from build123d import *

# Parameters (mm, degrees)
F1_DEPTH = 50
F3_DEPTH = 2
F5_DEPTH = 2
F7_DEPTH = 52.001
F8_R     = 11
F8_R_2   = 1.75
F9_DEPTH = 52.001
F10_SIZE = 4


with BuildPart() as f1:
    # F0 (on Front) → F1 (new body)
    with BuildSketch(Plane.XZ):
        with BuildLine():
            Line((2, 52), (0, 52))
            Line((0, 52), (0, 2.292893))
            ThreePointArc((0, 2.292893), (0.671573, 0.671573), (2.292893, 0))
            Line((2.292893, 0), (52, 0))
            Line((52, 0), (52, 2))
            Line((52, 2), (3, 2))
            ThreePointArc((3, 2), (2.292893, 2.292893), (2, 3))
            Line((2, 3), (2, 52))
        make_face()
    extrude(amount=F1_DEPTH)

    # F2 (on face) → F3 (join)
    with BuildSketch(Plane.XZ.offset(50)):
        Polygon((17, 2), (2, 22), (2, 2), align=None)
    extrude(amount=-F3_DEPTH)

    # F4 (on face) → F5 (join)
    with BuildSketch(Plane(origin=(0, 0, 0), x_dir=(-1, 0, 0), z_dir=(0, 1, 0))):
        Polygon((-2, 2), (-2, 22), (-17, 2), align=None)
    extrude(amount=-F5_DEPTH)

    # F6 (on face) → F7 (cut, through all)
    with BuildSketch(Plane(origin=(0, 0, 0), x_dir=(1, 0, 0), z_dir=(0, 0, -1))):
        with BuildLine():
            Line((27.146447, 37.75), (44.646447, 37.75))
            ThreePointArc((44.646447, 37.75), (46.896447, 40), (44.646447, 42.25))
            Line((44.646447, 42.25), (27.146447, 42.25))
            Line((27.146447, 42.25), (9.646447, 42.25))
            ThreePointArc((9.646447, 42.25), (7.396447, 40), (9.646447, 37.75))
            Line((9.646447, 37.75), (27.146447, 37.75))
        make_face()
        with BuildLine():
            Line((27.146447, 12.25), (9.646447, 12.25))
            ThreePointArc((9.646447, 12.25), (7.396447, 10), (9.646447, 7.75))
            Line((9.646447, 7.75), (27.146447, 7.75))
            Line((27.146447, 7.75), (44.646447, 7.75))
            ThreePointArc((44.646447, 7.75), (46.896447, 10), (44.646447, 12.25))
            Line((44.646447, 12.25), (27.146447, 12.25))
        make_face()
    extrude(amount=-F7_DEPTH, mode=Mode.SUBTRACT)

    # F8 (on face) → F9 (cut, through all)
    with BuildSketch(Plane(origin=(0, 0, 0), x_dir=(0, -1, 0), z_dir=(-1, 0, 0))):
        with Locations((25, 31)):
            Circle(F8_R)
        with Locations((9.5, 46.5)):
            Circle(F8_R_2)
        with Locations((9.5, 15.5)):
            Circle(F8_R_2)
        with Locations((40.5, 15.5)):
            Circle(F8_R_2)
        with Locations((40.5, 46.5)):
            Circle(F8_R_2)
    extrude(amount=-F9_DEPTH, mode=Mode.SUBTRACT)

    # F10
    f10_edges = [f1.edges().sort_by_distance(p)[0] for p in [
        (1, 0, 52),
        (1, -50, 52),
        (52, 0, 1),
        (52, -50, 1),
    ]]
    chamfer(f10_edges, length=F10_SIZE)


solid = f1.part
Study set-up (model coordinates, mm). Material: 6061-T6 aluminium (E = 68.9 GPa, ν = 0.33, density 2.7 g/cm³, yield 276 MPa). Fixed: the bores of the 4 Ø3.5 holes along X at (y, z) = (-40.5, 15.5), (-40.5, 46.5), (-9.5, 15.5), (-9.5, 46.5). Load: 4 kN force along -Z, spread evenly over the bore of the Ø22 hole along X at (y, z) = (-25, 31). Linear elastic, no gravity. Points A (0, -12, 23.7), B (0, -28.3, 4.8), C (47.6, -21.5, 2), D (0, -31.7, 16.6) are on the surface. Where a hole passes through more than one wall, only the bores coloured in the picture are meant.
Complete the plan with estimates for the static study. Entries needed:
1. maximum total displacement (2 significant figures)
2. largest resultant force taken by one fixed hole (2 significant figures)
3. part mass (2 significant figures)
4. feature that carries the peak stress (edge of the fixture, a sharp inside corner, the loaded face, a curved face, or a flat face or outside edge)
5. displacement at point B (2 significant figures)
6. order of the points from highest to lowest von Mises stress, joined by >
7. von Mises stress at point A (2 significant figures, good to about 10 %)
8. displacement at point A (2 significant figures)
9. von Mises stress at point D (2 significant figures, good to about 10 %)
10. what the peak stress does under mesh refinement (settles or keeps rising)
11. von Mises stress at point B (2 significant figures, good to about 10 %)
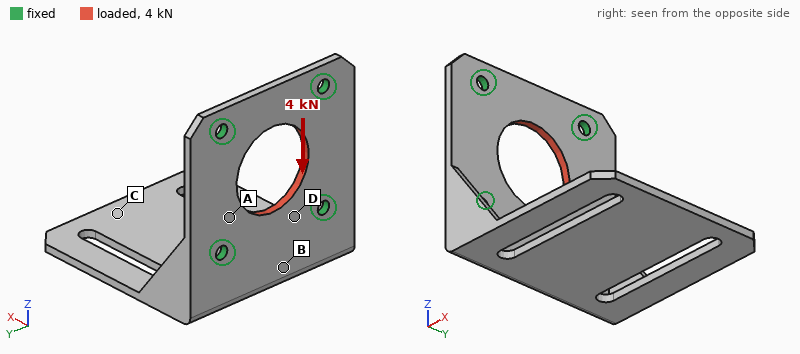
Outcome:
18 µm
1.0 kN
25 g
edge of the fixture
6.5 µm
A > D > B > C
41 MPa
4.4 µm
23 MPa
keeps rising
13 MPa
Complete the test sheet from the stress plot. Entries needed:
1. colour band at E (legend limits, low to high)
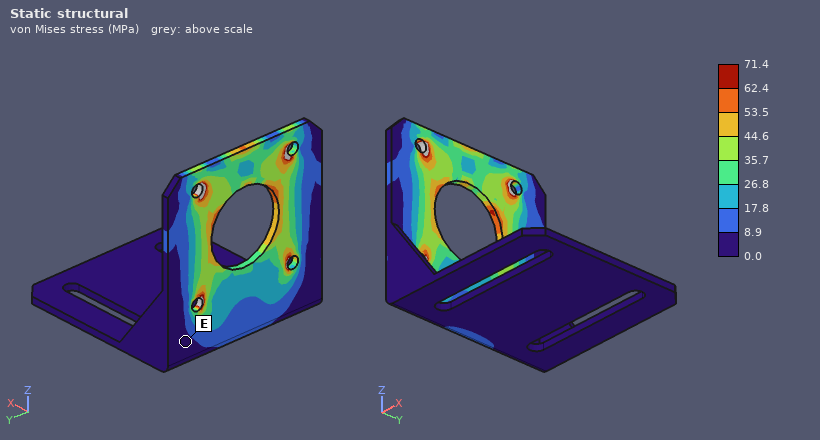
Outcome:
0.0 to 8.9 MPa
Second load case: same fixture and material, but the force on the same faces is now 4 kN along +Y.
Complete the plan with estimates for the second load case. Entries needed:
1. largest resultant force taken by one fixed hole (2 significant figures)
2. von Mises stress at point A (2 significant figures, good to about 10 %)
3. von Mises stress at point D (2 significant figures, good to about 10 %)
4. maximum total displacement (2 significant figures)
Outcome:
1.0 kN
31 MPa
36 MPa
14 µm
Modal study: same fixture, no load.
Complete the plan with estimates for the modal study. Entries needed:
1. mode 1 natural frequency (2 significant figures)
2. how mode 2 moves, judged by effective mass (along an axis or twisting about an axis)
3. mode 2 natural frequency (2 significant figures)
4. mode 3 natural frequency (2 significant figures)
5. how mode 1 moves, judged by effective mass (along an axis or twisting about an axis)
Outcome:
670 Hz
along Y
1400 Hz
2300 Hz
along Z
